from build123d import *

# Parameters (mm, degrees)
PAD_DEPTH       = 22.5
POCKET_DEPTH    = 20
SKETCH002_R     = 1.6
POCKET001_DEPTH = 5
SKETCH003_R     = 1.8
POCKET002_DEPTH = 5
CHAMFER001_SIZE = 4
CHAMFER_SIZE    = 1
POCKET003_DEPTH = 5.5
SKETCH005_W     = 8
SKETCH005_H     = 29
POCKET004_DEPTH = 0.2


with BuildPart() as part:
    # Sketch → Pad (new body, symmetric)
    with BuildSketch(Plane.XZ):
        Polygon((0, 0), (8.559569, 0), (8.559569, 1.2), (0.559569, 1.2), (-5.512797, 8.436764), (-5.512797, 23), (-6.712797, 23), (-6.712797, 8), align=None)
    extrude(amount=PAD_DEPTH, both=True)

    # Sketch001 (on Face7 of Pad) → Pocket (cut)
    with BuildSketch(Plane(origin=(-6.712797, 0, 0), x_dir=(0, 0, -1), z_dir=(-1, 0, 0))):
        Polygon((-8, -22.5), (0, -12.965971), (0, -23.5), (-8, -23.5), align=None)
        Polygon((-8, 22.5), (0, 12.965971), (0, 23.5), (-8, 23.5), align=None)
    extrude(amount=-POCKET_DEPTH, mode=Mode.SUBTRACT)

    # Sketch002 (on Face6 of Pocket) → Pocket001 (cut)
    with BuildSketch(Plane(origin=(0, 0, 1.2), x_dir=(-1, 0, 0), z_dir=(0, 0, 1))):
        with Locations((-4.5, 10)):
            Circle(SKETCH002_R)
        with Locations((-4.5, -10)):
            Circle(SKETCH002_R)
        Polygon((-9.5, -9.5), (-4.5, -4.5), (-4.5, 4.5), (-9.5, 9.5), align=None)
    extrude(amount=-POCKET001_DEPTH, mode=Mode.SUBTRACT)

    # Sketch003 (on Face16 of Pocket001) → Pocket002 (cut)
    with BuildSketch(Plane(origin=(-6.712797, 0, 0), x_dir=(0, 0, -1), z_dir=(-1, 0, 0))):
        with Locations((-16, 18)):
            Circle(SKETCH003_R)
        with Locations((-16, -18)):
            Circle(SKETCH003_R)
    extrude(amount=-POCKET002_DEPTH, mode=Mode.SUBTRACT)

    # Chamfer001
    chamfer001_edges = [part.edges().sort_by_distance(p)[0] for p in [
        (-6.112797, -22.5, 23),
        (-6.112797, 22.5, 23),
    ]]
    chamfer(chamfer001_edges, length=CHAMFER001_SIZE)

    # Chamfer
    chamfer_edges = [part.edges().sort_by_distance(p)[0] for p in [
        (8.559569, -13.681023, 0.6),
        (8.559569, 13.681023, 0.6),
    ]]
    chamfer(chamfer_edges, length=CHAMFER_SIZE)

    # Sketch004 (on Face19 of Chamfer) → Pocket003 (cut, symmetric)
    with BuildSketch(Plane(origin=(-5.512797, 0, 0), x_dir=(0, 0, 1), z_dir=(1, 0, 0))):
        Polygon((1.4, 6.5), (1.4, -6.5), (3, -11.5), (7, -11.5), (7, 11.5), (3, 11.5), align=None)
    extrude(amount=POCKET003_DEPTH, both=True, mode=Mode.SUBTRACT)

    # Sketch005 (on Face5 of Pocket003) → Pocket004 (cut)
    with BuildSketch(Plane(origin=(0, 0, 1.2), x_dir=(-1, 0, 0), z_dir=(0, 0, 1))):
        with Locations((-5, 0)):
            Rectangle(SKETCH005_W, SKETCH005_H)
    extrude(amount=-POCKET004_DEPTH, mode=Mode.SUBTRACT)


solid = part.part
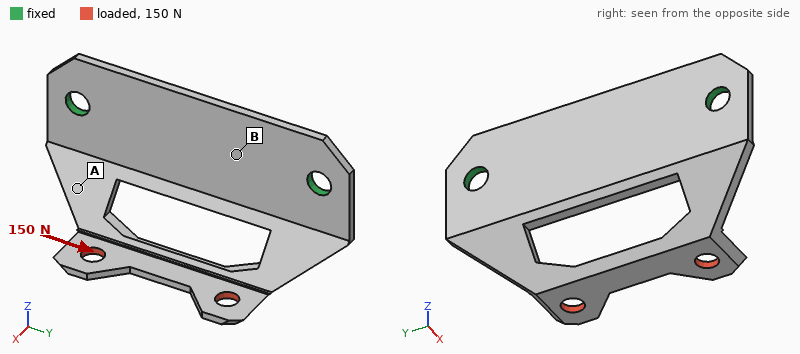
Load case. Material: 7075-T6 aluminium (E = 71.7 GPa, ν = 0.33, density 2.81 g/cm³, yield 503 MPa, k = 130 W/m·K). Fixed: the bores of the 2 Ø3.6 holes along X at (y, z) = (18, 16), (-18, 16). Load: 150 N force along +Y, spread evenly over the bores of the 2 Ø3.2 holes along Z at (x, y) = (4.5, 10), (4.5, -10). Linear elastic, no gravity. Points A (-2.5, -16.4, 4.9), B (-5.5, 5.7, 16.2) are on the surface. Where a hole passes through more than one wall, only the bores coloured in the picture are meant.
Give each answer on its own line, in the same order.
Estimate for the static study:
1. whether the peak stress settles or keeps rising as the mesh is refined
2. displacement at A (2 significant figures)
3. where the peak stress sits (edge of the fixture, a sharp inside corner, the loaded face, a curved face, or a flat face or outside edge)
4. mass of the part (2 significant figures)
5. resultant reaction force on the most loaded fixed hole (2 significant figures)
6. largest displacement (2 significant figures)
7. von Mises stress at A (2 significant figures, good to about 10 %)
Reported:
keeps rising
0.085 mm
edge of the fixture
3.3 g
100 N
0.22 mm
30 MPa
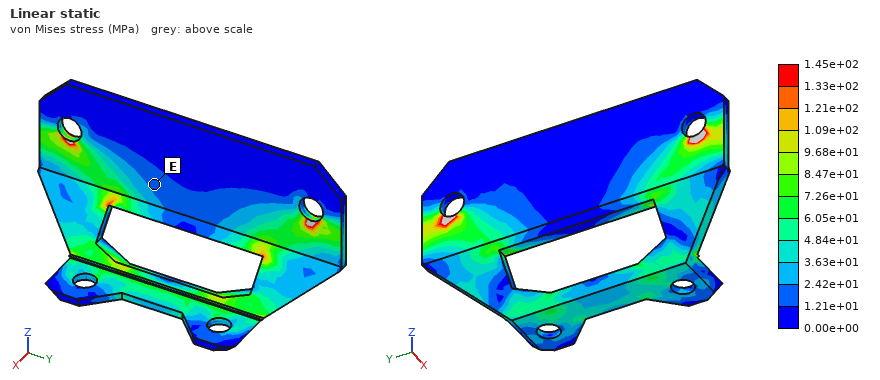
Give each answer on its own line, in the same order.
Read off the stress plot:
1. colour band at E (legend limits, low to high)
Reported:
1.21e+01 to 2.42e+01 MPa
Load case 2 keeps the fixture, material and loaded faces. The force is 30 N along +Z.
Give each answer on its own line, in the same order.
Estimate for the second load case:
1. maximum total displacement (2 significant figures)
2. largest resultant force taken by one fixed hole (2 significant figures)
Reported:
0.38 mm
16 N
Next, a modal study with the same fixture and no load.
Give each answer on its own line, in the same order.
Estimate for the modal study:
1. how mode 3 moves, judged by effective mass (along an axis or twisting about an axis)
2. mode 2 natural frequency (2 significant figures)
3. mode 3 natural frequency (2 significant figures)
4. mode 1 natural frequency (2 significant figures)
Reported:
along X
4300 Hz
6000 Hz
2100 Hz
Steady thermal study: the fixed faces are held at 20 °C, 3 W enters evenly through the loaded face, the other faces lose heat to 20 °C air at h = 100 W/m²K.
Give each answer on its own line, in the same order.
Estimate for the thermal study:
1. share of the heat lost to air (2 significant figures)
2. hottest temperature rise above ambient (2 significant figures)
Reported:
44 %
23 K
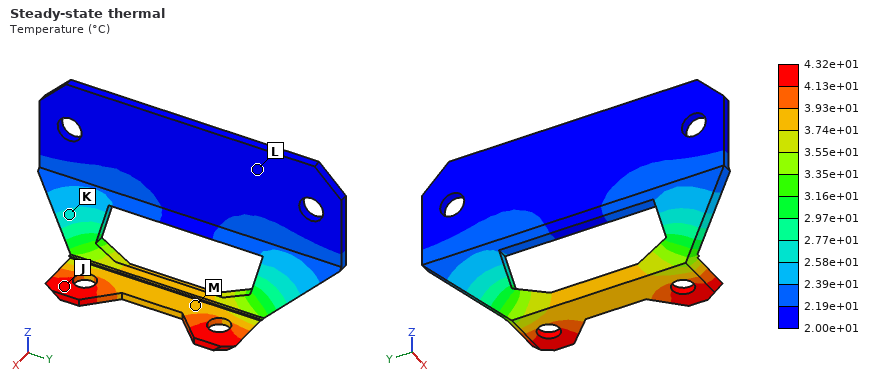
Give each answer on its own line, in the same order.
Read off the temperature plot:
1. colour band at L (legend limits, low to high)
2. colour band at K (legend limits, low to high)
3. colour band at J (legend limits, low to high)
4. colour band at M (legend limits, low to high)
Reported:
2.00e+01 to 2.19e+01 °C
2.58e+01 to 2.77e+01 °C
4.13e+01 to 4.32e+01 °C
3.74e+01 to 3.93e+01 °C
